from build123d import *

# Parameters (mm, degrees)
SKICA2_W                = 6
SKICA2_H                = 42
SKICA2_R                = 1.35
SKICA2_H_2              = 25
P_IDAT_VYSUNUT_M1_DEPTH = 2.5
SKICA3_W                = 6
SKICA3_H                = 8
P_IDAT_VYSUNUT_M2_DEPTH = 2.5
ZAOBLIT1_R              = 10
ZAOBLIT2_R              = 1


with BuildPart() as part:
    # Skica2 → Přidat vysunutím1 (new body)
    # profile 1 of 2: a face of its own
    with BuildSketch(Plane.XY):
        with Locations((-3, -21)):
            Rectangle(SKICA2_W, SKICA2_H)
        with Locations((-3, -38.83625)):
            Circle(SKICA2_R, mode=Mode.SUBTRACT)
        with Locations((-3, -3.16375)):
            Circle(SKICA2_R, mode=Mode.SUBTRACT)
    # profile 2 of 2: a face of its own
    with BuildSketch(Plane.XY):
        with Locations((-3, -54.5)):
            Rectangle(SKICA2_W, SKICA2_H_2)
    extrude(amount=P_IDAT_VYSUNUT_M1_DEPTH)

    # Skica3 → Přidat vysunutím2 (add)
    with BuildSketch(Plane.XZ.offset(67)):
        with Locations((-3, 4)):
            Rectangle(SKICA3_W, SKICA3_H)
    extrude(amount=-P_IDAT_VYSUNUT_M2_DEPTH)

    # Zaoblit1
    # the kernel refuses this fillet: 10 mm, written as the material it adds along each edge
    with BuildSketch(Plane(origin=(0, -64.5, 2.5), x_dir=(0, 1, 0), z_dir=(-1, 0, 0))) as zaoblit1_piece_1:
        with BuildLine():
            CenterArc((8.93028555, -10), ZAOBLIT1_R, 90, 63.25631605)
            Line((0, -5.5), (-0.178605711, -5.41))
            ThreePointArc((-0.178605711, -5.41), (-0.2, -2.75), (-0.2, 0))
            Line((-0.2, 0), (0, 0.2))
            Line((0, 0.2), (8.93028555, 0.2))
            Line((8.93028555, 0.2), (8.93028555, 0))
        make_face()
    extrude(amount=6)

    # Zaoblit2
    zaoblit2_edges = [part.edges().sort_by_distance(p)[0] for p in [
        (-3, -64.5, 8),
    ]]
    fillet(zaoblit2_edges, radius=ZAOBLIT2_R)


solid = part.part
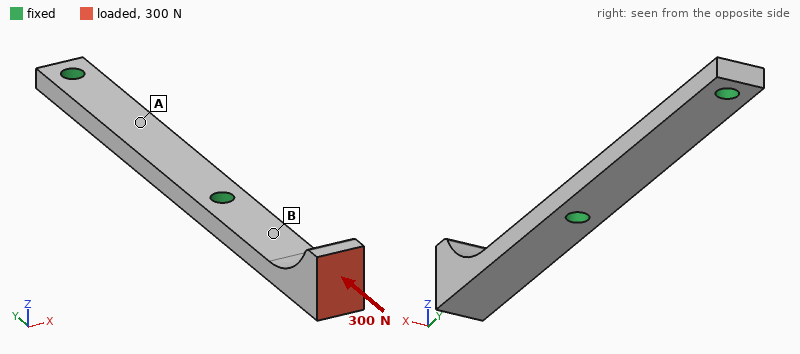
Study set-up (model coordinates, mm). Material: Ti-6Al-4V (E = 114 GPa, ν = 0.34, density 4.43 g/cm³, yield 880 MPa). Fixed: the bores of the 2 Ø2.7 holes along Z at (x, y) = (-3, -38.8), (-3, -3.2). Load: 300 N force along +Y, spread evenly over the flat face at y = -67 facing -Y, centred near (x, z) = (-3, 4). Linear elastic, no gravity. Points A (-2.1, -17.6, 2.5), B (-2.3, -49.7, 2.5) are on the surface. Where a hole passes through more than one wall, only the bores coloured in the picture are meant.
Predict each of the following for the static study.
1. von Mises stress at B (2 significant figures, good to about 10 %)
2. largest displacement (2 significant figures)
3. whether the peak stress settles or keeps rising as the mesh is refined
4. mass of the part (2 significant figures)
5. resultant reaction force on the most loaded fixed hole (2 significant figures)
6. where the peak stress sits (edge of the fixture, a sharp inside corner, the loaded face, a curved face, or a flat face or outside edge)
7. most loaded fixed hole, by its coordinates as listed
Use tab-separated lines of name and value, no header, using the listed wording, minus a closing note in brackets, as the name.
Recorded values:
von Mises stress at B	150 MPa
largest displacement	0.34 mm
whether the peak stress settles or keeps rising as the mesh is refined	keeps rising
mass of the part	5.1 g
resultant reaction force on the most loaded fixed hole	300 N
where the peak stress sits	edge of the fixture
most loaded fixed hole, by its coordinates as listed	(-3, -38.8)
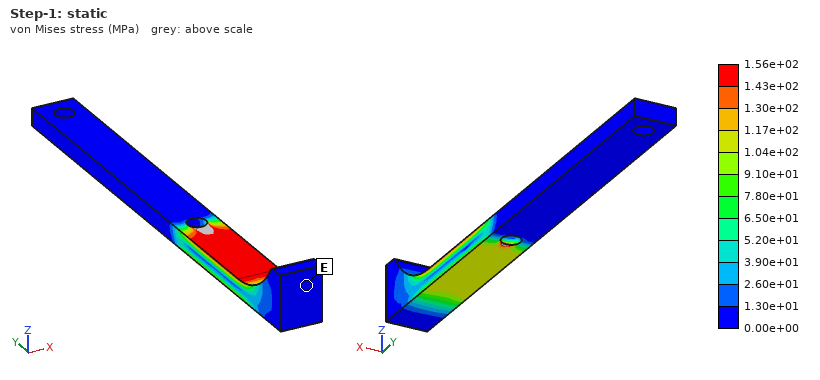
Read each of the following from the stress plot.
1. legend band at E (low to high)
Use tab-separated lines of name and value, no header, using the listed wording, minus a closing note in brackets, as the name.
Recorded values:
legend band at E	0.00e+00 to 1.30e+01 MPa
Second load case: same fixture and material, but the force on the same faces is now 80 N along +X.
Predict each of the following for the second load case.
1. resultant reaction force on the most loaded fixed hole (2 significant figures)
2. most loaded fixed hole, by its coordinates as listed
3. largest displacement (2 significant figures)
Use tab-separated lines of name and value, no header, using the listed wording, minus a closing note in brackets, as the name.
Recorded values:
resultant reaction force on the most loaded fixed hole	89 N
most loaded fixed hole, by its coordinates as listed	(-3, -38.8)
largest displacement	0.16 mm
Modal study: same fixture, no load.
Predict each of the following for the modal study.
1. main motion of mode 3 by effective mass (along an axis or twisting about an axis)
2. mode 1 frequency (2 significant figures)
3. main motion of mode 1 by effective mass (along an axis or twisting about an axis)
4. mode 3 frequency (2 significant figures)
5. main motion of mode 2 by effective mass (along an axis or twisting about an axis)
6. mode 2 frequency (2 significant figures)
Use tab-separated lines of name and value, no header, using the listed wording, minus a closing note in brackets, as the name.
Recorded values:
main motion of mode 3 by effective mass	along Z
mode 1 frequency	1800 Hz
main motion of mode 1 by effective mass	along Z
mode 3 frequency	11 kHz
main motion of mode 2 by effective mass	along X
mode 2 frequency	3800 Hz
